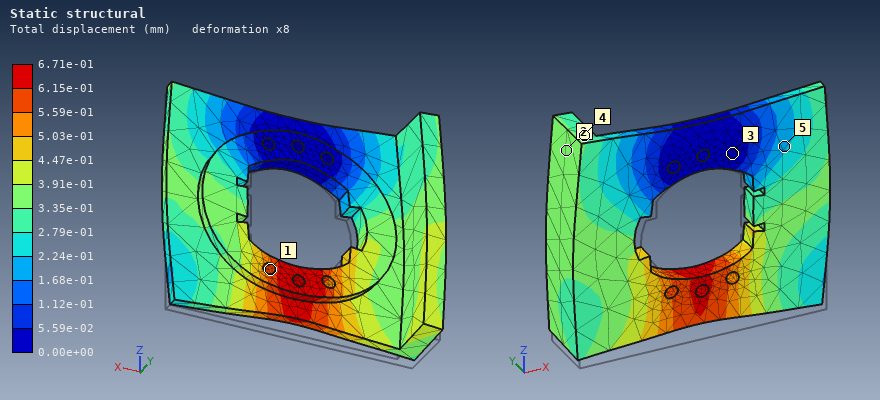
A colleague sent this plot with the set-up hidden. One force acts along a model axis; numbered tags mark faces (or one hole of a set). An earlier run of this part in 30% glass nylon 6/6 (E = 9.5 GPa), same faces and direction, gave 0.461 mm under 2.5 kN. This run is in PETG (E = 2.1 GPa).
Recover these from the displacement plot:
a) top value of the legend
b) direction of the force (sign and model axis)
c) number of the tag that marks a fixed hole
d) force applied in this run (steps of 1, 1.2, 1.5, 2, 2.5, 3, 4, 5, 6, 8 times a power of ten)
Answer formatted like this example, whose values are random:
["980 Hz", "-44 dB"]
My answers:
["6.71e-01 mm", "+Z", "3", "800 N"]
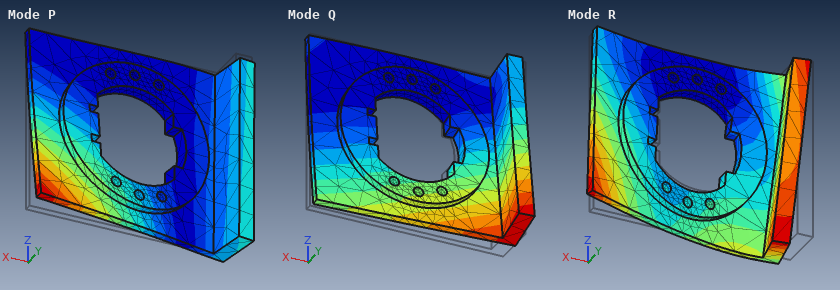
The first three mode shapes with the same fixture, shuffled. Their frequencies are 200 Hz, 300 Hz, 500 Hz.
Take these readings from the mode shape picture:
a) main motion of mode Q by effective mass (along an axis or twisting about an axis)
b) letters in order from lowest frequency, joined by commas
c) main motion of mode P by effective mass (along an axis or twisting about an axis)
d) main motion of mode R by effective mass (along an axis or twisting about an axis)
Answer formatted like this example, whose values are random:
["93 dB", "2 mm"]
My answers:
["along Y", "Q, P, R", "twisting about Z", "along X"]
